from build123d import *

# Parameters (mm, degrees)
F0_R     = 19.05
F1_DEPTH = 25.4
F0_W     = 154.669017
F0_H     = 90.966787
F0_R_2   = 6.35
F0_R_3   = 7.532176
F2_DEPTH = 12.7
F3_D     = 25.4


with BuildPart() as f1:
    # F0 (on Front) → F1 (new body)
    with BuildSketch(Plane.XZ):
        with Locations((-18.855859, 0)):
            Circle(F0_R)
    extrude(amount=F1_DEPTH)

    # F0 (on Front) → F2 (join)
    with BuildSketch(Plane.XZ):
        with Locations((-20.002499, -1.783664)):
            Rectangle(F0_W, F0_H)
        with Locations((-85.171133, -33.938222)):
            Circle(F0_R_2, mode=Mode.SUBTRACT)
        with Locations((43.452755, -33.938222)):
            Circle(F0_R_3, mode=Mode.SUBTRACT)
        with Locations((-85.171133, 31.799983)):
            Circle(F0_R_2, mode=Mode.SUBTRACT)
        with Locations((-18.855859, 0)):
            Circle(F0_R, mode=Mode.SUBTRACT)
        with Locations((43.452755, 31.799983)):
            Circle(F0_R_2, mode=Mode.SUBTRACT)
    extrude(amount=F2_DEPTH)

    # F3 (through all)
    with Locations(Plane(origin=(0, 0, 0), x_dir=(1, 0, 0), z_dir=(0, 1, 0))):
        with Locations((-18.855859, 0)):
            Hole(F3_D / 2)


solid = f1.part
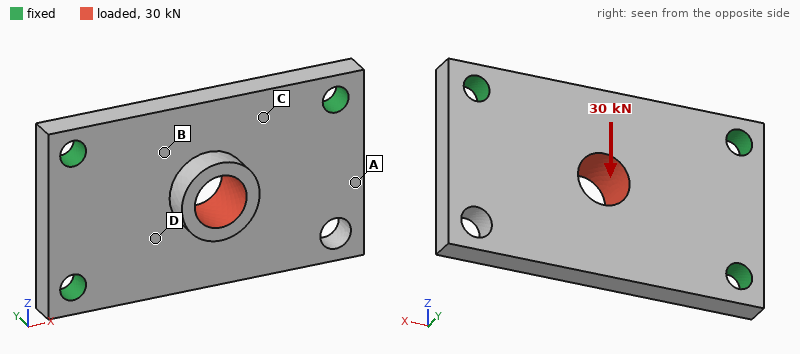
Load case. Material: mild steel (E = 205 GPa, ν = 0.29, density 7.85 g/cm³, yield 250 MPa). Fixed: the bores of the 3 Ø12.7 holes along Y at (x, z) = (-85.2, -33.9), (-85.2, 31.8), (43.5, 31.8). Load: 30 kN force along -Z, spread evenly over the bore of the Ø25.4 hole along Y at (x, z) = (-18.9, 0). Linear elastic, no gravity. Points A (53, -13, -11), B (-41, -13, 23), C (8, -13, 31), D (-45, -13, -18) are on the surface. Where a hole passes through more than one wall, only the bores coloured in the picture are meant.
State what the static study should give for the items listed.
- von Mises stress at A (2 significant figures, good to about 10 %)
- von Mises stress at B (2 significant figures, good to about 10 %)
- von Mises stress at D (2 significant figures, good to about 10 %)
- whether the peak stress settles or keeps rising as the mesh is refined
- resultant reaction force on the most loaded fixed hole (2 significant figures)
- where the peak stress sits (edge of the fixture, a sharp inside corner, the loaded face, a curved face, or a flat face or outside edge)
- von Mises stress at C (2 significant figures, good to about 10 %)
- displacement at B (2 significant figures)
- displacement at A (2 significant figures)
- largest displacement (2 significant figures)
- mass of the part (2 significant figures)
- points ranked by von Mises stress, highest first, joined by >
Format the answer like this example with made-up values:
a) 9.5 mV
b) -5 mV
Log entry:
a) 17 MPa
b) 49 MPa
c) 60 MPa
d) keeps rising
e) 14 kN
f) edge of the fixture
g) 35 MPa
h) 17 µm
i) 20 µm
j) 56 µm
k) 1.4 kg
l) D > B > C > A
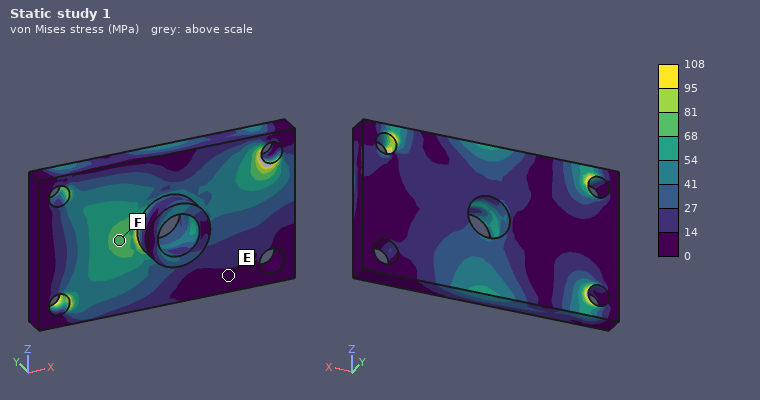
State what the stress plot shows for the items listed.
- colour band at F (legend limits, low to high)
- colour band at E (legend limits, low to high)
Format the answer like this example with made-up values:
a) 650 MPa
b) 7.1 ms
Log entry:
a) 68 to 81 MPa
b) 0 to 14 MPa
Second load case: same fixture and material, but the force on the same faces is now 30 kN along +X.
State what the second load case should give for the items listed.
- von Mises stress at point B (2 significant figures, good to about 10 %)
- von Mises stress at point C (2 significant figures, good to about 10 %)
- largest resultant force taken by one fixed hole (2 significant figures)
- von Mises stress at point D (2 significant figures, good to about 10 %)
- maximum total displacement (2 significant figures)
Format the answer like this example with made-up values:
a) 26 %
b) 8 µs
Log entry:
a) 37 MPa
b) 28 MPa
c) 11 kN
d) 39 MPa
e) 27 µm
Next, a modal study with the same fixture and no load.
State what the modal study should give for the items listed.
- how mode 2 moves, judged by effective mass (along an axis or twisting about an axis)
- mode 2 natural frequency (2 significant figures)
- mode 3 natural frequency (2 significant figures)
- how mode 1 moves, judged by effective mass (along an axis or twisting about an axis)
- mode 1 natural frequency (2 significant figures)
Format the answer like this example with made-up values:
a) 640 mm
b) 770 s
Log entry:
a) along Y
b) 3900 Hz
c) 5400 Hz
d) along Y
e) 2000 Hz
